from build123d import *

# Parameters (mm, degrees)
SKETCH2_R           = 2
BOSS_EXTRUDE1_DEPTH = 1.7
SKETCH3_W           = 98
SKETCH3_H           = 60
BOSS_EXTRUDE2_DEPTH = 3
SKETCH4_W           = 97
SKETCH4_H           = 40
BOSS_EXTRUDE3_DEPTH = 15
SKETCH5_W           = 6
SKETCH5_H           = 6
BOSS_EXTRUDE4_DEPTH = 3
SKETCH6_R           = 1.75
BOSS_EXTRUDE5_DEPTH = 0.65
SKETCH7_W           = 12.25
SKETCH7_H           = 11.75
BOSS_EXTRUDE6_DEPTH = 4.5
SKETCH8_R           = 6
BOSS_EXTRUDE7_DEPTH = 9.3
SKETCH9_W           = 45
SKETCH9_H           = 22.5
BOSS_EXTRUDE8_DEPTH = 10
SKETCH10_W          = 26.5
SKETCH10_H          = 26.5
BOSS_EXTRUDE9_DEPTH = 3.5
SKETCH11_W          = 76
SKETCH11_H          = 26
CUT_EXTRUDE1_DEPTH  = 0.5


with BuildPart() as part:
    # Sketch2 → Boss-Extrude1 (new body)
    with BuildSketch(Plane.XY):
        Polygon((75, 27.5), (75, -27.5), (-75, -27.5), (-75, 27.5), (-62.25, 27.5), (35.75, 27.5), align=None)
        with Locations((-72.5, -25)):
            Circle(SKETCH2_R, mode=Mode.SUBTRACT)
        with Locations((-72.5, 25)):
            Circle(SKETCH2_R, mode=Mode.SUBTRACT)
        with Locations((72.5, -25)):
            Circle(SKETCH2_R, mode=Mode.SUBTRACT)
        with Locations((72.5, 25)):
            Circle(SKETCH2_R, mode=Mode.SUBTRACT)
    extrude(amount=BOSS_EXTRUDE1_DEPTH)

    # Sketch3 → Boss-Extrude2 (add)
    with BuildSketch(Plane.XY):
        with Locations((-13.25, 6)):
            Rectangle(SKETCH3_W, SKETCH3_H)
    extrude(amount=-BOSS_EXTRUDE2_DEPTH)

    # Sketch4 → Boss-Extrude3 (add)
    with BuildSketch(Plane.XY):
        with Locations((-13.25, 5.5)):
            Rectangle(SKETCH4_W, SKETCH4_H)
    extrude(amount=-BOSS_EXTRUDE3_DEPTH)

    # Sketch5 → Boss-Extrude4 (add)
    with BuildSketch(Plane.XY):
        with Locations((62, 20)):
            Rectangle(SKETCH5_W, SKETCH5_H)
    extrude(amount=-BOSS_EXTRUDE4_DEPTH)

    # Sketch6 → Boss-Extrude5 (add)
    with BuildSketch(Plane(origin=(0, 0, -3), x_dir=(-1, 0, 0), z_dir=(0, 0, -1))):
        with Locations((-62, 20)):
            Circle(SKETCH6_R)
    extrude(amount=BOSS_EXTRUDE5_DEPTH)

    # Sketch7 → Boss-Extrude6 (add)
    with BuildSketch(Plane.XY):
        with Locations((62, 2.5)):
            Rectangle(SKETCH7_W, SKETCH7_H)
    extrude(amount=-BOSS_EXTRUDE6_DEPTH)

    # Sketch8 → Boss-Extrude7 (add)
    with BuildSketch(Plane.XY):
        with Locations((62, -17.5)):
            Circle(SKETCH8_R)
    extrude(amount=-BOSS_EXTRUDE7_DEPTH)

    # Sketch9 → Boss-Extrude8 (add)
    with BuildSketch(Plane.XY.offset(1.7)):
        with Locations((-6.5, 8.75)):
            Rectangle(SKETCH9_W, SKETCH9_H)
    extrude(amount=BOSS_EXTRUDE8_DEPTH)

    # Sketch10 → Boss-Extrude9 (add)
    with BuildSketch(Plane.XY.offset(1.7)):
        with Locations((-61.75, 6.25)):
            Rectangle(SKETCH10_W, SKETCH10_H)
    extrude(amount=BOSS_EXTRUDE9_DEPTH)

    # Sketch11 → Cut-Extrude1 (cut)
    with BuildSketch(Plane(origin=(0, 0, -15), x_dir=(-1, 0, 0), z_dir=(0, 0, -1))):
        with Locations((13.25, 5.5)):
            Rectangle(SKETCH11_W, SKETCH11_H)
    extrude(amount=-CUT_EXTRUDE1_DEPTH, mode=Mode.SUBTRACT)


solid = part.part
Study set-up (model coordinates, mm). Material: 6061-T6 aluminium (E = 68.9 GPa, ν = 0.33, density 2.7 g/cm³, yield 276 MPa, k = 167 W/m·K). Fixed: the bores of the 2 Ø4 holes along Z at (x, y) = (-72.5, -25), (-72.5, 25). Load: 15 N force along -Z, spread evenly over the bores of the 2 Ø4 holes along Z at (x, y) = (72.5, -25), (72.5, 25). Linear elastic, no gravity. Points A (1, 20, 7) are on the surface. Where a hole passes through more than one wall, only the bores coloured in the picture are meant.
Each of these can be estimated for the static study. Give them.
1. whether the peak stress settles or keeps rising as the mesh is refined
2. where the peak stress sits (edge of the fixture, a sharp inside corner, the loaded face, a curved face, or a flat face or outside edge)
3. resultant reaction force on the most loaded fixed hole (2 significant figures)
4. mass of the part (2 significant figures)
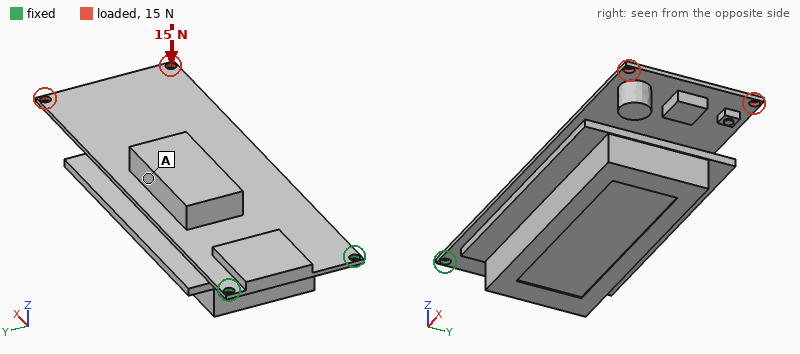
keeps rising
edge of the fixture
47 N
250 g
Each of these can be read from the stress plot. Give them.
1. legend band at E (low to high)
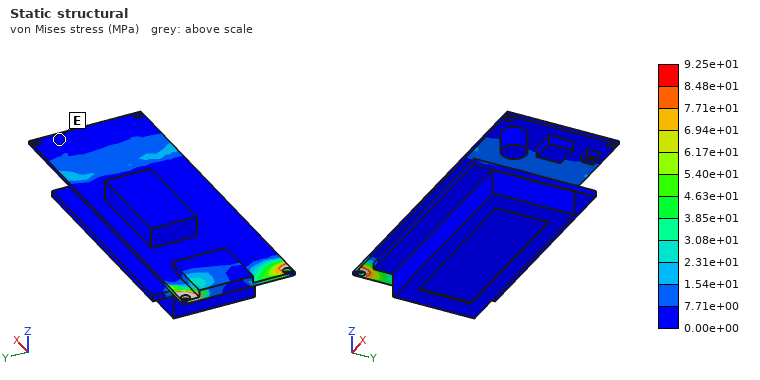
0.00e+00 to 7.71e+00 MPa
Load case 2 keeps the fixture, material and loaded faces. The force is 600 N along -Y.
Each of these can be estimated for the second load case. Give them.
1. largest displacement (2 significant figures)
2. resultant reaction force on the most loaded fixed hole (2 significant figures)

0.25 mm
1.8 kN
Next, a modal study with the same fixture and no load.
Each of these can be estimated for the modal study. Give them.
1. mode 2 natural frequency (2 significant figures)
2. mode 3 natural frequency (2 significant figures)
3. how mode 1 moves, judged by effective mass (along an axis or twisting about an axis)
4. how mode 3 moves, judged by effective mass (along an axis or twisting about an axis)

770 Hz
1200 Hz
along Z
along Y
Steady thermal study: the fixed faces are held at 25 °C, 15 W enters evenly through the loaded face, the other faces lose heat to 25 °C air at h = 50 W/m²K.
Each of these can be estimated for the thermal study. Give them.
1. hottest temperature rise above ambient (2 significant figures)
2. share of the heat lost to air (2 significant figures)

68 K
79 %
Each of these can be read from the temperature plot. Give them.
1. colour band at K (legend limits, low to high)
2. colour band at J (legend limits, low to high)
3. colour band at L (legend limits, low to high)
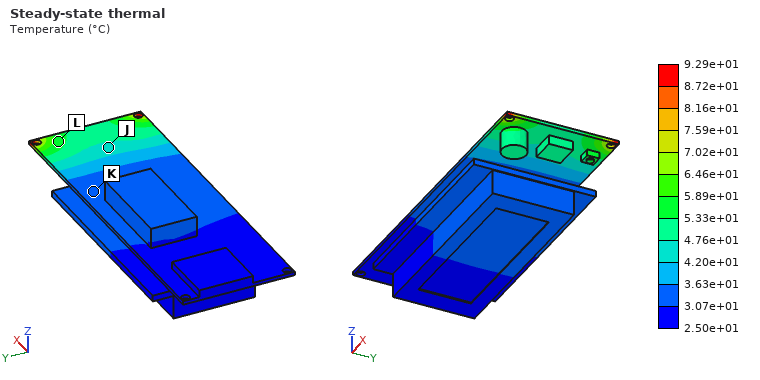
3.07e+01 to 3.63e+01 °C
4.20e+01 to 4.76e+01 °C
5.33e+01 to 5.89e+01 °C
